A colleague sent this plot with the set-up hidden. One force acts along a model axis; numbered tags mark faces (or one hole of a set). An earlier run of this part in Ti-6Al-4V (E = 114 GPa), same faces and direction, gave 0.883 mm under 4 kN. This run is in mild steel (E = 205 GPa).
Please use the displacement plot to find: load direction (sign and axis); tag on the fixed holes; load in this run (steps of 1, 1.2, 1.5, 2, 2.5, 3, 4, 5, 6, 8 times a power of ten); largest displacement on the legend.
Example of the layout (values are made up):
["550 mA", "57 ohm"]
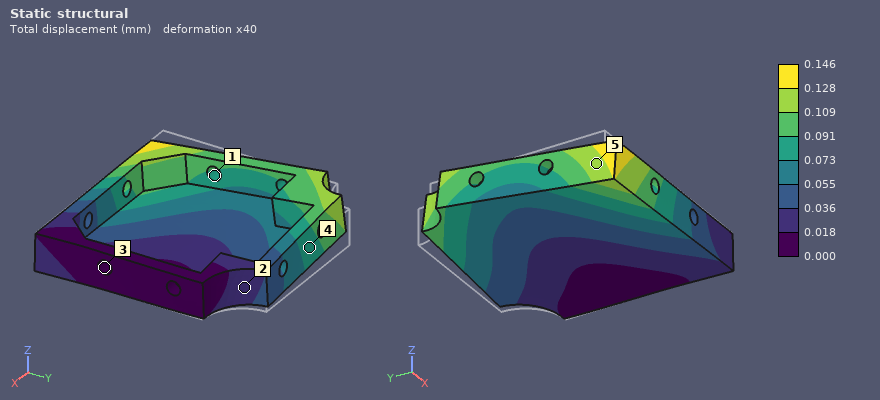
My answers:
["-Y", "3", "1.2 kN", "0.146 mm"]
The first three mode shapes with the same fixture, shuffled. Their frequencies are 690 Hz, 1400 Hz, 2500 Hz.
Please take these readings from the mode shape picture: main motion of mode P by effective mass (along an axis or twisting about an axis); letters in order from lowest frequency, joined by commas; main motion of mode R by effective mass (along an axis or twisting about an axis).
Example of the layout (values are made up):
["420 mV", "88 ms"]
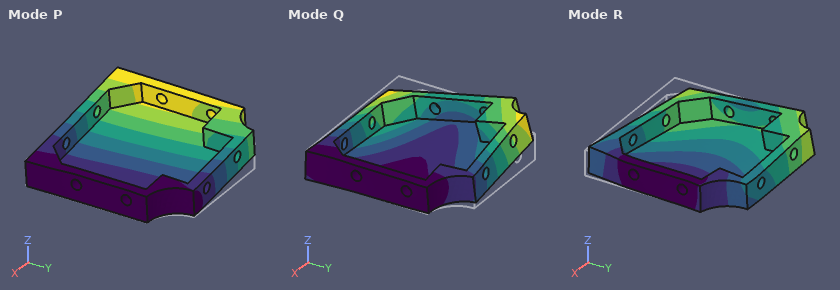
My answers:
["along Z", "P, Q, R", "along Y"]
